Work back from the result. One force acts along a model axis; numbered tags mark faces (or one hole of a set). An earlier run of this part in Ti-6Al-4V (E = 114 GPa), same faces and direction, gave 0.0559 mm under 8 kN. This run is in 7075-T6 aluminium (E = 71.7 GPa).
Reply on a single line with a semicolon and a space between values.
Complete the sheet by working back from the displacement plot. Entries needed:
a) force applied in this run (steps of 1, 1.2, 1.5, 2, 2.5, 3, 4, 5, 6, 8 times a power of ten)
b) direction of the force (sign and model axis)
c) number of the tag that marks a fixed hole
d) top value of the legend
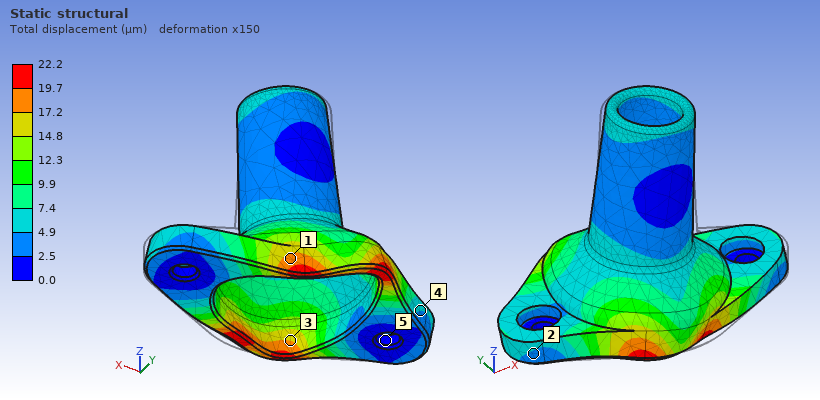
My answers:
2 kN; -X; 5; 22.2 µm
